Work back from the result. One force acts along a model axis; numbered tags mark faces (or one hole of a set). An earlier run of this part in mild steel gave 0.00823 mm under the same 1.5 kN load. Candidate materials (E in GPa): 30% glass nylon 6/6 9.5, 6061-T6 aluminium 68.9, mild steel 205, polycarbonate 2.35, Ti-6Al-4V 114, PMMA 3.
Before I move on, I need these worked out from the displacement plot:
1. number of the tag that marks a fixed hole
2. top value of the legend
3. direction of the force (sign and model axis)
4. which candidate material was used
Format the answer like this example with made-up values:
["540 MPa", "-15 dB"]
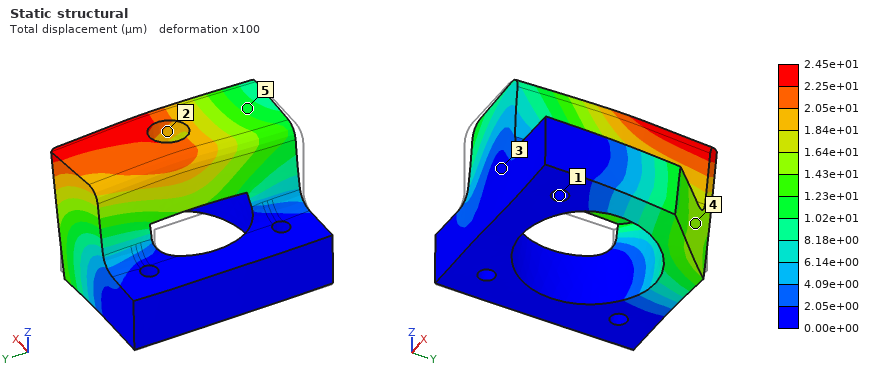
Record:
["1", "2.45e+01 µm", "+X", "6061-T6 aluminium"]
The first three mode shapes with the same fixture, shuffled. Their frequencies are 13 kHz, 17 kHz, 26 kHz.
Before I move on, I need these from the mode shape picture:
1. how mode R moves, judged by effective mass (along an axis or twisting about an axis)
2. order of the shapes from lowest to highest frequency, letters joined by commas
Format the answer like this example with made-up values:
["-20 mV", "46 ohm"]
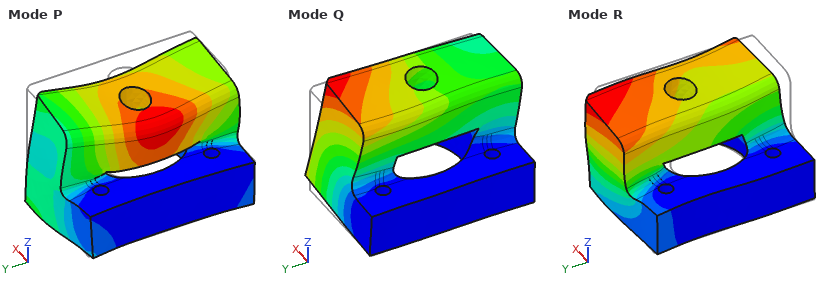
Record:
["along Y", "Q, R, P"]
